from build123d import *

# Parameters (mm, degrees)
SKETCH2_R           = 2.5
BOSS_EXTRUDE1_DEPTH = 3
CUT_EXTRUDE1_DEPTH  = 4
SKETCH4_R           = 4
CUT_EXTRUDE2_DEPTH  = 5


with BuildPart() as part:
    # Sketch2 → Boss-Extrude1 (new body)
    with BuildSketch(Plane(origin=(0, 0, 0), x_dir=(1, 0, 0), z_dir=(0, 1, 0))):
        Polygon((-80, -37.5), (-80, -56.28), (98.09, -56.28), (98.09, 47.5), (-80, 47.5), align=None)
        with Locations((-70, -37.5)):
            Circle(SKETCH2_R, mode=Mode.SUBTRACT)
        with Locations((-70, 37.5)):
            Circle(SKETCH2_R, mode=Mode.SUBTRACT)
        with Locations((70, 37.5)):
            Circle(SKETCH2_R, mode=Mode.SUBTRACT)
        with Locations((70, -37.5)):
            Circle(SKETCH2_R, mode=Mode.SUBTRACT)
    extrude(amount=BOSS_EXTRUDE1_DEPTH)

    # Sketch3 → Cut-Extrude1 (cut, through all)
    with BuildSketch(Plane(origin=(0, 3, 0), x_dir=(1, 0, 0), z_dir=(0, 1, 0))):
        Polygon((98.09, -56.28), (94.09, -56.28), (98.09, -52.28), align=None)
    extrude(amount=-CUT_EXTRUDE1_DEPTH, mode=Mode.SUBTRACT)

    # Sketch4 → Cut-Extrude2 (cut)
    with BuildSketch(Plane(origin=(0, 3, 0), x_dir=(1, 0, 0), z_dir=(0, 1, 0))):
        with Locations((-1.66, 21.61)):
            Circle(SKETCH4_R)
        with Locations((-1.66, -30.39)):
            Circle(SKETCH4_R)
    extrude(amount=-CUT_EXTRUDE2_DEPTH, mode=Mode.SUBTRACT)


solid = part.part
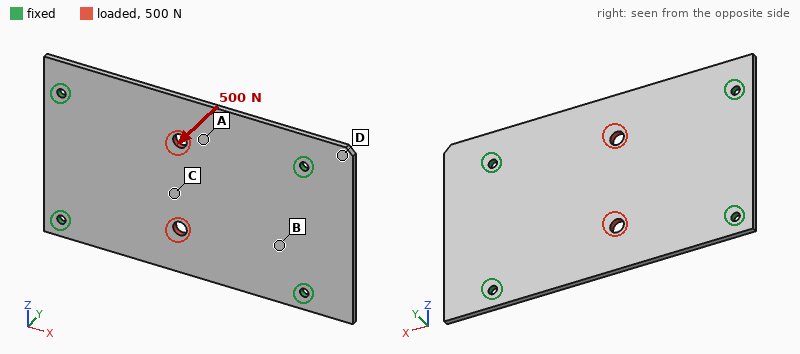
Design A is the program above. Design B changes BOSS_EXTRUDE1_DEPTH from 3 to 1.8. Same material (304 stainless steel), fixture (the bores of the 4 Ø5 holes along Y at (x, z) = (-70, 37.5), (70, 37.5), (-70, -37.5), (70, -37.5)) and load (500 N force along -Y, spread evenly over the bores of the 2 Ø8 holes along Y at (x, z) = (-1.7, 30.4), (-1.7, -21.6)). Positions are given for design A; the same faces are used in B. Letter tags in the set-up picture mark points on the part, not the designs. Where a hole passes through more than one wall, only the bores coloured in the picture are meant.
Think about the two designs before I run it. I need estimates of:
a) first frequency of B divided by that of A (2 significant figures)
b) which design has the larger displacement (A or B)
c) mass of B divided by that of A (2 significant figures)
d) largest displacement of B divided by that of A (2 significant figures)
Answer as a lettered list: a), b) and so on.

a) 0.61
b) B
c) 0.60
d) 4.5
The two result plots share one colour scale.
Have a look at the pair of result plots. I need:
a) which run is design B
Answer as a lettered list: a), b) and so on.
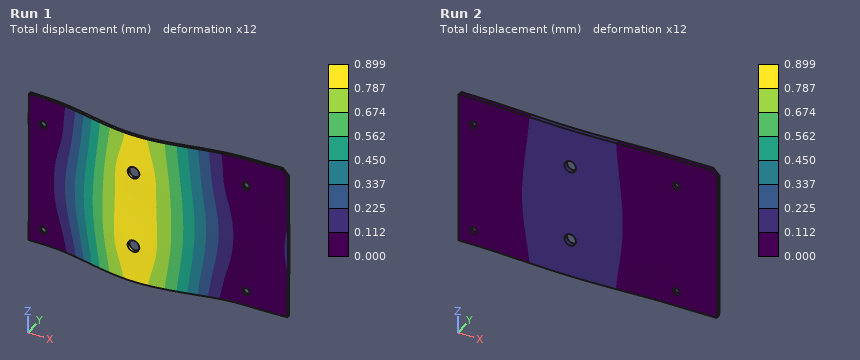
a) Run 1
